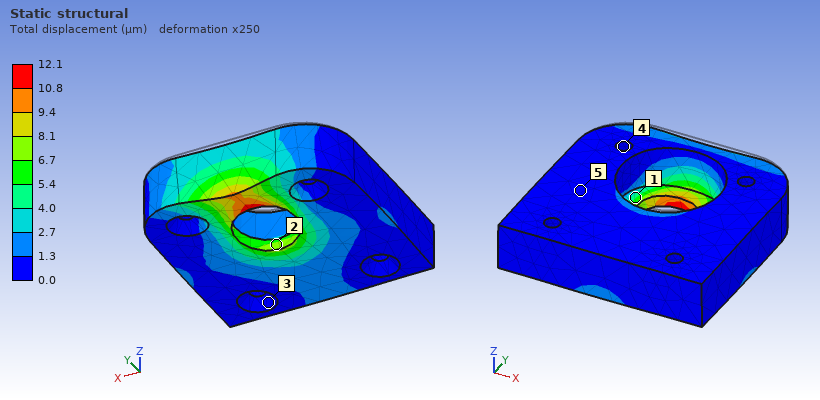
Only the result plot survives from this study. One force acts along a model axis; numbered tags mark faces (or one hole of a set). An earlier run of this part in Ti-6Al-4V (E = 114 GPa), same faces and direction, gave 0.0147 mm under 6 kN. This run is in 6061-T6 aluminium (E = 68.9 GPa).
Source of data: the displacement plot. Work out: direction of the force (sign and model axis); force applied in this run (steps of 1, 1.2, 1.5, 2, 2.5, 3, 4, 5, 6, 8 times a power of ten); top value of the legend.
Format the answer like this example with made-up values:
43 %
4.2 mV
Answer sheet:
-Y
3 kN
12.1 µm
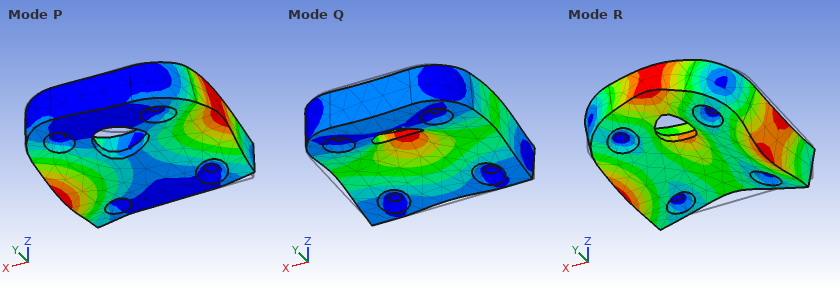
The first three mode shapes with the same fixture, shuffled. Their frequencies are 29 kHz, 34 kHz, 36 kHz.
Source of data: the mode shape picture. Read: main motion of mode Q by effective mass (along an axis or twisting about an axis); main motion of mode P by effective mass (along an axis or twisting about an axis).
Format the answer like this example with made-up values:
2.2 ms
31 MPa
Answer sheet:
along Z
twisting about Y
